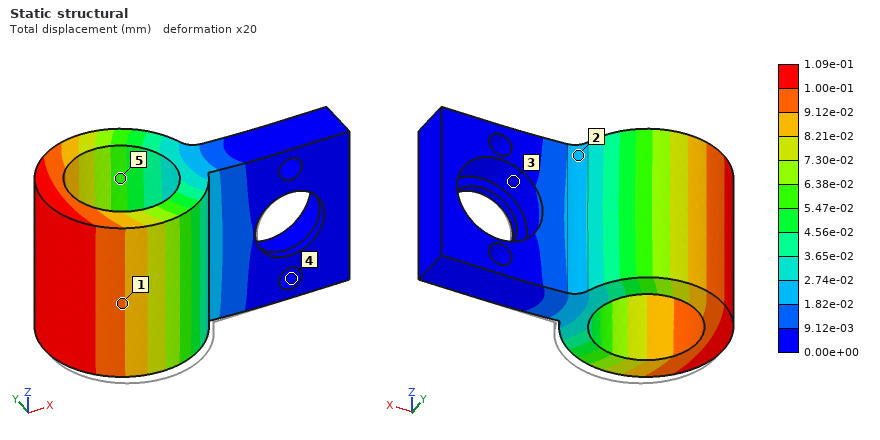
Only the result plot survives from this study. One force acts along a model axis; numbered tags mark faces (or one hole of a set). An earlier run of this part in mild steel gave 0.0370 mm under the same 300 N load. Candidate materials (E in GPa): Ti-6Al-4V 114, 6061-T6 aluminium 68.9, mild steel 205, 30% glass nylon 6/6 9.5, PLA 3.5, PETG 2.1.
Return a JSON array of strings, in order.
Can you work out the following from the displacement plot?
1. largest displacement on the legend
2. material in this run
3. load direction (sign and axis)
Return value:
["1.09e-01 mm", "6061-T6 aluminium", "+Y"]
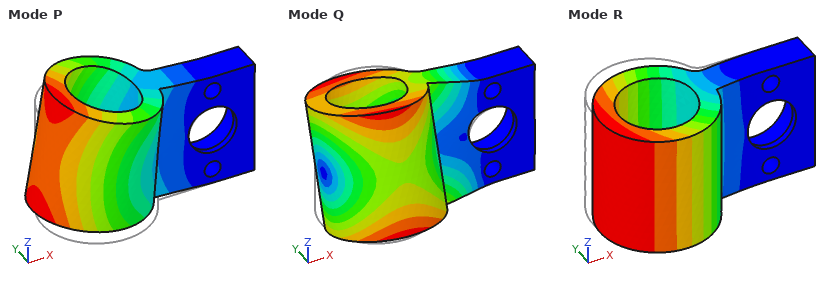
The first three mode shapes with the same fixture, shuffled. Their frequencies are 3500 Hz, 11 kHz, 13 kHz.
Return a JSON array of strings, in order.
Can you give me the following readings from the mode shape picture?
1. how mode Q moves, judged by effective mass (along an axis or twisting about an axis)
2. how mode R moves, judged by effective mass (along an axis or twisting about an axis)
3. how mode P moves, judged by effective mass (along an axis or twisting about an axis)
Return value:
["twisting about X", "along Y", "along Z"]
